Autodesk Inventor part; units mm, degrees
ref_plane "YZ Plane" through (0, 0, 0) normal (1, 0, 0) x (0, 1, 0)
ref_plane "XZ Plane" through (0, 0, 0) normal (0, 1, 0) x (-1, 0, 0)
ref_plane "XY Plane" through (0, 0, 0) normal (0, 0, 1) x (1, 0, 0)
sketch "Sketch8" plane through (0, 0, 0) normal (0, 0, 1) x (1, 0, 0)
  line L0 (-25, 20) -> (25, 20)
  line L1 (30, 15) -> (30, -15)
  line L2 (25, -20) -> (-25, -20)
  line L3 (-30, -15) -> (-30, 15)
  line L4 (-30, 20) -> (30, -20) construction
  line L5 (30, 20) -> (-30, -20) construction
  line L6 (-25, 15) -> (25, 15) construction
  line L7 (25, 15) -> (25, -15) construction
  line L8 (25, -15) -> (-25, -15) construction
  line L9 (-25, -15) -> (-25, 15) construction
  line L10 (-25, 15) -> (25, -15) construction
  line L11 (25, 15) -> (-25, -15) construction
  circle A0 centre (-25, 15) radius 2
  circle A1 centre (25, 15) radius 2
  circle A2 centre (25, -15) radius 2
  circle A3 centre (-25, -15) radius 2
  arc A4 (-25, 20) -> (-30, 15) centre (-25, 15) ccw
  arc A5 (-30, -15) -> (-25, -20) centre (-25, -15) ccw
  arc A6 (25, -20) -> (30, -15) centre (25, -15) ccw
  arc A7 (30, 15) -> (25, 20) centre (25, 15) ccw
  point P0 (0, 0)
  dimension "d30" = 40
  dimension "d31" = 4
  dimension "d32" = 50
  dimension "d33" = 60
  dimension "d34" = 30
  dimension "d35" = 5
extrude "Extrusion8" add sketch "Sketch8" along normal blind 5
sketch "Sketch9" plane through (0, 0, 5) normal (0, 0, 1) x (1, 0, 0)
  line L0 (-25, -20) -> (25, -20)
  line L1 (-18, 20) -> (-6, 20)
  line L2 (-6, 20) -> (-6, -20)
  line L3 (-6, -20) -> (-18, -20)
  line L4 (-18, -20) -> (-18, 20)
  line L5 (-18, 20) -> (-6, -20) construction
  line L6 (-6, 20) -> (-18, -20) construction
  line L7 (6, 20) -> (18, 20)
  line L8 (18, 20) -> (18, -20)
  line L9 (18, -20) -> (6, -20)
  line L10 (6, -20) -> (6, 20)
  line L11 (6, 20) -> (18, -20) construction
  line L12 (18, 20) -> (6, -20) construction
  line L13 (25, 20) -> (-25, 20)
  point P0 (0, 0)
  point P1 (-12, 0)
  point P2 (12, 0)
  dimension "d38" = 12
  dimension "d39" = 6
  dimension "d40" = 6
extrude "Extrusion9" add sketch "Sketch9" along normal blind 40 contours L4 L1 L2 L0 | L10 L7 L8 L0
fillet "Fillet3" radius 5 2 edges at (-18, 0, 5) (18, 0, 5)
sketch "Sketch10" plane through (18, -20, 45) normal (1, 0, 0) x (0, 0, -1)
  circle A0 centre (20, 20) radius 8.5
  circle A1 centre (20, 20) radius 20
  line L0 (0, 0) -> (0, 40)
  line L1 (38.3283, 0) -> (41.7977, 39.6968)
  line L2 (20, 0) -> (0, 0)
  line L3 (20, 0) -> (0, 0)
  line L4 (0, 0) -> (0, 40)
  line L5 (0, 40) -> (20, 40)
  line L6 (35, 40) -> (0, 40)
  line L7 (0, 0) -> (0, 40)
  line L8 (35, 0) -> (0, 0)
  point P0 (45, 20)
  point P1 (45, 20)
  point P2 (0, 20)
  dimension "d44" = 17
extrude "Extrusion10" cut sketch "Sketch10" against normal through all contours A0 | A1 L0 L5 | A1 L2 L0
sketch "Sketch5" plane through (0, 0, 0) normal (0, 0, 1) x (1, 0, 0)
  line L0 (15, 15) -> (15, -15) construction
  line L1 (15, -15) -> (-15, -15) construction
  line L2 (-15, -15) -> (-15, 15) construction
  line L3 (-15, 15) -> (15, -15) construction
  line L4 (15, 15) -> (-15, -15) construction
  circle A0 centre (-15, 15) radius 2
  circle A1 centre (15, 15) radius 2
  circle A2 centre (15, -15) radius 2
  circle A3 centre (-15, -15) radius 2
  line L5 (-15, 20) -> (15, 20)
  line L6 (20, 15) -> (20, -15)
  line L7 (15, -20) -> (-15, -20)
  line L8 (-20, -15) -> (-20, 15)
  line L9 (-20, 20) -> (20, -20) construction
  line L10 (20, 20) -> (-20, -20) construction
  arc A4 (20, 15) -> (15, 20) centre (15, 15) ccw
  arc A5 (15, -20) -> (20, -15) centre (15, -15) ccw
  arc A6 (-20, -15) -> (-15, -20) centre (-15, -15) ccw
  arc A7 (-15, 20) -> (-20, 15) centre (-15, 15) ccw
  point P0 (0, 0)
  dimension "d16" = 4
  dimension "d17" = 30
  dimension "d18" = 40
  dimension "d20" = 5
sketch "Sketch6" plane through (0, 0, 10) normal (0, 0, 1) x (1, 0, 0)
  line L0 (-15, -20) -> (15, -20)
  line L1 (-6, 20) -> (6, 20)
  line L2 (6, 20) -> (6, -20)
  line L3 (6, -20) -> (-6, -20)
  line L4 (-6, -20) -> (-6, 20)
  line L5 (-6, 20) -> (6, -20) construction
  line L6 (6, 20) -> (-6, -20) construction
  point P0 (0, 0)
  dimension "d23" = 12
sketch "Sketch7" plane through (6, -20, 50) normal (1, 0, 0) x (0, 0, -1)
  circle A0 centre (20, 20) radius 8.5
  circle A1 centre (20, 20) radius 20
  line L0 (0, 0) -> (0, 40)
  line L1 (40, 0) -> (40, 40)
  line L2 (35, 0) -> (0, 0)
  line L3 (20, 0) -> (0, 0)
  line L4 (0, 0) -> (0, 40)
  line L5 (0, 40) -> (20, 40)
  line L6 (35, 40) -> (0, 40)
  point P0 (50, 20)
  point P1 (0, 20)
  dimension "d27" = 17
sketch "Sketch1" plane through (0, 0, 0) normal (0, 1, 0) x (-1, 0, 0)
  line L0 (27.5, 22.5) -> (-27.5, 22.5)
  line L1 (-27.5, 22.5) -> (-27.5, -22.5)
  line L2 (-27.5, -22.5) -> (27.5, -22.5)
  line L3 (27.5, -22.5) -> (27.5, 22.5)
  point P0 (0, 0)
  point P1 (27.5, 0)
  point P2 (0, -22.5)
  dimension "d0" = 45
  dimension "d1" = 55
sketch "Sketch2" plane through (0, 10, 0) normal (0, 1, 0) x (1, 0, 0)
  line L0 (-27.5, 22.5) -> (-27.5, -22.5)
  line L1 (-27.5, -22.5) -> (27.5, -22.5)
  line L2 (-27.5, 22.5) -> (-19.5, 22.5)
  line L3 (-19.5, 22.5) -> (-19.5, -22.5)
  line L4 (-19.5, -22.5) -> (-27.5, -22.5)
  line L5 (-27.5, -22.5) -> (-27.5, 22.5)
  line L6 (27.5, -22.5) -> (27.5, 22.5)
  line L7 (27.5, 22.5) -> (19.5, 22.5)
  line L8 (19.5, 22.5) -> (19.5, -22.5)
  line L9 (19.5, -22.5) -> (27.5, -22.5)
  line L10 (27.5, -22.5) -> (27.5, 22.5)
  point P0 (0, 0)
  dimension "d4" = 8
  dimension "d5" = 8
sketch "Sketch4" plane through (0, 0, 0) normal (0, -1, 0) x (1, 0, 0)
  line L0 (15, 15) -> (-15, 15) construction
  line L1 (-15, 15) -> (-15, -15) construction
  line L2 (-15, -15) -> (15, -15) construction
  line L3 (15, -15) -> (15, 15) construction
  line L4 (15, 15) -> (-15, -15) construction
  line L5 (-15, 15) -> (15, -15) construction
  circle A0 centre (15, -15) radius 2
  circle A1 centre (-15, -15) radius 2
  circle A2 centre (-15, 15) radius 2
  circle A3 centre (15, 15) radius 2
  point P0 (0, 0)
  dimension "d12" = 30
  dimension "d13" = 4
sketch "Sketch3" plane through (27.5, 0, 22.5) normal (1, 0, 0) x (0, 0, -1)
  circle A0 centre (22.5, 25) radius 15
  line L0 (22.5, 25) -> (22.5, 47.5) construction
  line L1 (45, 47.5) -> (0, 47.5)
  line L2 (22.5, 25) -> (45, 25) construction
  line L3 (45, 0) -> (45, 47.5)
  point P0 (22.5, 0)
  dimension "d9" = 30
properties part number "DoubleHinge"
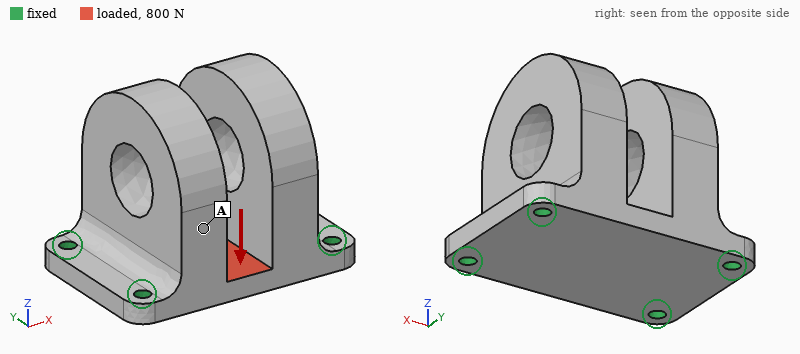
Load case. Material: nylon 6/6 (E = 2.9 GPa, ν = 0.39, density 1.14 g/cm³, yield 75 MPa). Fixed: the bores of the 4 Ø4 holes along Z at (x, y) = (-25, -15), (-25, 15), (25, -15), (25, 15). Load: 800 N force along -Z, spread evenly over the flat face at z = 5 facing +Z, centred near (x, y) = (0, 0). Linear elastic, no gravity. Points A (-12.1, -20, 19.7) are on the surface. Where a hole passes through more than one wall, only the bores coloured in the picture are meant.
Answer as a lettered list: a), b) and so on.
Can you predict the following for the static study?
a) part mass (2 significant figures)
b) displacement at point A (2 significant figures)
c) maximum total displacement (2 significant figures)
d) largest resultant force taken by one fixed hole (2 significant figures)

a) 47 g
b) 0.43 mm
c) 0.98 mm
d) 200 N
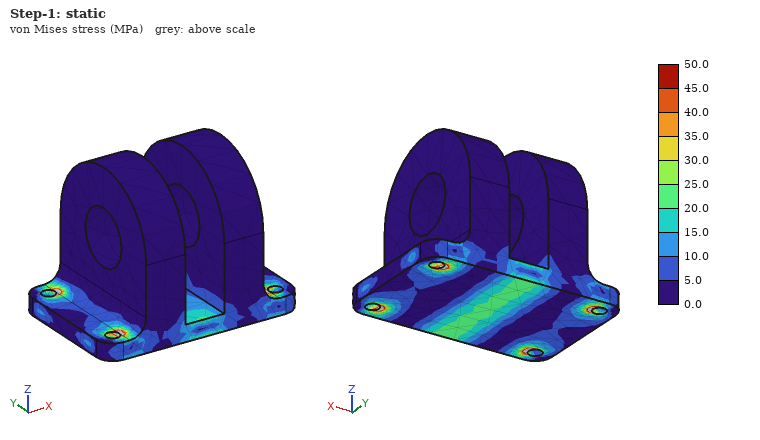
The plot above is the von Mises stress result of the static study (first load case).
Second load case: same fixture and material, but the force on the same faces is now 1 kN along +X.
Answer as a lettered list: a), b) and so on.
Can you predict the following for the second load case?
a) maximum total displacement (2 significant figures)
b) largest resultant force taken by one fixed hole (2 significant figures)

a) 29 µm
b) 260 N
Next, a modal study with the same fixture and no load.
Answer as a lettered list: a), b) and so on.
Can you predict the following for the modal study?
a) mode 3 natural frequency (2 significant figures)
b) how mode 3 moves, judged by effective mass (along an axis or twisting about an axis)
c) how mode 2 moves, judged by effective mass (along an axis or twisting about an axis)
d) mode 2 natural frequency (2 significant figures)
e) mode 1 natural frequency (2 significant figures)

a) 1700 Hz
b) along Y
c) along X
d) 1600 Hz
e) 800 Hz
